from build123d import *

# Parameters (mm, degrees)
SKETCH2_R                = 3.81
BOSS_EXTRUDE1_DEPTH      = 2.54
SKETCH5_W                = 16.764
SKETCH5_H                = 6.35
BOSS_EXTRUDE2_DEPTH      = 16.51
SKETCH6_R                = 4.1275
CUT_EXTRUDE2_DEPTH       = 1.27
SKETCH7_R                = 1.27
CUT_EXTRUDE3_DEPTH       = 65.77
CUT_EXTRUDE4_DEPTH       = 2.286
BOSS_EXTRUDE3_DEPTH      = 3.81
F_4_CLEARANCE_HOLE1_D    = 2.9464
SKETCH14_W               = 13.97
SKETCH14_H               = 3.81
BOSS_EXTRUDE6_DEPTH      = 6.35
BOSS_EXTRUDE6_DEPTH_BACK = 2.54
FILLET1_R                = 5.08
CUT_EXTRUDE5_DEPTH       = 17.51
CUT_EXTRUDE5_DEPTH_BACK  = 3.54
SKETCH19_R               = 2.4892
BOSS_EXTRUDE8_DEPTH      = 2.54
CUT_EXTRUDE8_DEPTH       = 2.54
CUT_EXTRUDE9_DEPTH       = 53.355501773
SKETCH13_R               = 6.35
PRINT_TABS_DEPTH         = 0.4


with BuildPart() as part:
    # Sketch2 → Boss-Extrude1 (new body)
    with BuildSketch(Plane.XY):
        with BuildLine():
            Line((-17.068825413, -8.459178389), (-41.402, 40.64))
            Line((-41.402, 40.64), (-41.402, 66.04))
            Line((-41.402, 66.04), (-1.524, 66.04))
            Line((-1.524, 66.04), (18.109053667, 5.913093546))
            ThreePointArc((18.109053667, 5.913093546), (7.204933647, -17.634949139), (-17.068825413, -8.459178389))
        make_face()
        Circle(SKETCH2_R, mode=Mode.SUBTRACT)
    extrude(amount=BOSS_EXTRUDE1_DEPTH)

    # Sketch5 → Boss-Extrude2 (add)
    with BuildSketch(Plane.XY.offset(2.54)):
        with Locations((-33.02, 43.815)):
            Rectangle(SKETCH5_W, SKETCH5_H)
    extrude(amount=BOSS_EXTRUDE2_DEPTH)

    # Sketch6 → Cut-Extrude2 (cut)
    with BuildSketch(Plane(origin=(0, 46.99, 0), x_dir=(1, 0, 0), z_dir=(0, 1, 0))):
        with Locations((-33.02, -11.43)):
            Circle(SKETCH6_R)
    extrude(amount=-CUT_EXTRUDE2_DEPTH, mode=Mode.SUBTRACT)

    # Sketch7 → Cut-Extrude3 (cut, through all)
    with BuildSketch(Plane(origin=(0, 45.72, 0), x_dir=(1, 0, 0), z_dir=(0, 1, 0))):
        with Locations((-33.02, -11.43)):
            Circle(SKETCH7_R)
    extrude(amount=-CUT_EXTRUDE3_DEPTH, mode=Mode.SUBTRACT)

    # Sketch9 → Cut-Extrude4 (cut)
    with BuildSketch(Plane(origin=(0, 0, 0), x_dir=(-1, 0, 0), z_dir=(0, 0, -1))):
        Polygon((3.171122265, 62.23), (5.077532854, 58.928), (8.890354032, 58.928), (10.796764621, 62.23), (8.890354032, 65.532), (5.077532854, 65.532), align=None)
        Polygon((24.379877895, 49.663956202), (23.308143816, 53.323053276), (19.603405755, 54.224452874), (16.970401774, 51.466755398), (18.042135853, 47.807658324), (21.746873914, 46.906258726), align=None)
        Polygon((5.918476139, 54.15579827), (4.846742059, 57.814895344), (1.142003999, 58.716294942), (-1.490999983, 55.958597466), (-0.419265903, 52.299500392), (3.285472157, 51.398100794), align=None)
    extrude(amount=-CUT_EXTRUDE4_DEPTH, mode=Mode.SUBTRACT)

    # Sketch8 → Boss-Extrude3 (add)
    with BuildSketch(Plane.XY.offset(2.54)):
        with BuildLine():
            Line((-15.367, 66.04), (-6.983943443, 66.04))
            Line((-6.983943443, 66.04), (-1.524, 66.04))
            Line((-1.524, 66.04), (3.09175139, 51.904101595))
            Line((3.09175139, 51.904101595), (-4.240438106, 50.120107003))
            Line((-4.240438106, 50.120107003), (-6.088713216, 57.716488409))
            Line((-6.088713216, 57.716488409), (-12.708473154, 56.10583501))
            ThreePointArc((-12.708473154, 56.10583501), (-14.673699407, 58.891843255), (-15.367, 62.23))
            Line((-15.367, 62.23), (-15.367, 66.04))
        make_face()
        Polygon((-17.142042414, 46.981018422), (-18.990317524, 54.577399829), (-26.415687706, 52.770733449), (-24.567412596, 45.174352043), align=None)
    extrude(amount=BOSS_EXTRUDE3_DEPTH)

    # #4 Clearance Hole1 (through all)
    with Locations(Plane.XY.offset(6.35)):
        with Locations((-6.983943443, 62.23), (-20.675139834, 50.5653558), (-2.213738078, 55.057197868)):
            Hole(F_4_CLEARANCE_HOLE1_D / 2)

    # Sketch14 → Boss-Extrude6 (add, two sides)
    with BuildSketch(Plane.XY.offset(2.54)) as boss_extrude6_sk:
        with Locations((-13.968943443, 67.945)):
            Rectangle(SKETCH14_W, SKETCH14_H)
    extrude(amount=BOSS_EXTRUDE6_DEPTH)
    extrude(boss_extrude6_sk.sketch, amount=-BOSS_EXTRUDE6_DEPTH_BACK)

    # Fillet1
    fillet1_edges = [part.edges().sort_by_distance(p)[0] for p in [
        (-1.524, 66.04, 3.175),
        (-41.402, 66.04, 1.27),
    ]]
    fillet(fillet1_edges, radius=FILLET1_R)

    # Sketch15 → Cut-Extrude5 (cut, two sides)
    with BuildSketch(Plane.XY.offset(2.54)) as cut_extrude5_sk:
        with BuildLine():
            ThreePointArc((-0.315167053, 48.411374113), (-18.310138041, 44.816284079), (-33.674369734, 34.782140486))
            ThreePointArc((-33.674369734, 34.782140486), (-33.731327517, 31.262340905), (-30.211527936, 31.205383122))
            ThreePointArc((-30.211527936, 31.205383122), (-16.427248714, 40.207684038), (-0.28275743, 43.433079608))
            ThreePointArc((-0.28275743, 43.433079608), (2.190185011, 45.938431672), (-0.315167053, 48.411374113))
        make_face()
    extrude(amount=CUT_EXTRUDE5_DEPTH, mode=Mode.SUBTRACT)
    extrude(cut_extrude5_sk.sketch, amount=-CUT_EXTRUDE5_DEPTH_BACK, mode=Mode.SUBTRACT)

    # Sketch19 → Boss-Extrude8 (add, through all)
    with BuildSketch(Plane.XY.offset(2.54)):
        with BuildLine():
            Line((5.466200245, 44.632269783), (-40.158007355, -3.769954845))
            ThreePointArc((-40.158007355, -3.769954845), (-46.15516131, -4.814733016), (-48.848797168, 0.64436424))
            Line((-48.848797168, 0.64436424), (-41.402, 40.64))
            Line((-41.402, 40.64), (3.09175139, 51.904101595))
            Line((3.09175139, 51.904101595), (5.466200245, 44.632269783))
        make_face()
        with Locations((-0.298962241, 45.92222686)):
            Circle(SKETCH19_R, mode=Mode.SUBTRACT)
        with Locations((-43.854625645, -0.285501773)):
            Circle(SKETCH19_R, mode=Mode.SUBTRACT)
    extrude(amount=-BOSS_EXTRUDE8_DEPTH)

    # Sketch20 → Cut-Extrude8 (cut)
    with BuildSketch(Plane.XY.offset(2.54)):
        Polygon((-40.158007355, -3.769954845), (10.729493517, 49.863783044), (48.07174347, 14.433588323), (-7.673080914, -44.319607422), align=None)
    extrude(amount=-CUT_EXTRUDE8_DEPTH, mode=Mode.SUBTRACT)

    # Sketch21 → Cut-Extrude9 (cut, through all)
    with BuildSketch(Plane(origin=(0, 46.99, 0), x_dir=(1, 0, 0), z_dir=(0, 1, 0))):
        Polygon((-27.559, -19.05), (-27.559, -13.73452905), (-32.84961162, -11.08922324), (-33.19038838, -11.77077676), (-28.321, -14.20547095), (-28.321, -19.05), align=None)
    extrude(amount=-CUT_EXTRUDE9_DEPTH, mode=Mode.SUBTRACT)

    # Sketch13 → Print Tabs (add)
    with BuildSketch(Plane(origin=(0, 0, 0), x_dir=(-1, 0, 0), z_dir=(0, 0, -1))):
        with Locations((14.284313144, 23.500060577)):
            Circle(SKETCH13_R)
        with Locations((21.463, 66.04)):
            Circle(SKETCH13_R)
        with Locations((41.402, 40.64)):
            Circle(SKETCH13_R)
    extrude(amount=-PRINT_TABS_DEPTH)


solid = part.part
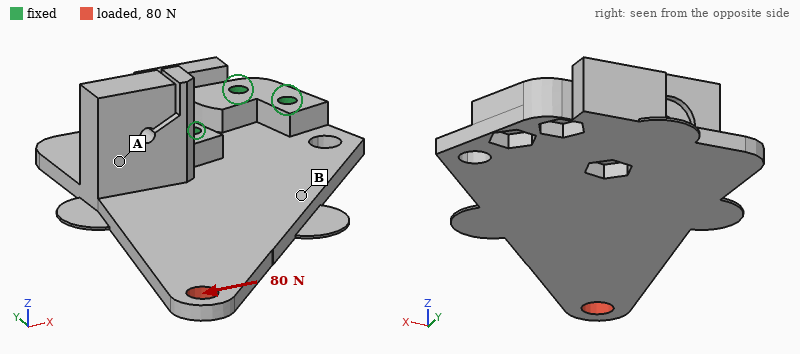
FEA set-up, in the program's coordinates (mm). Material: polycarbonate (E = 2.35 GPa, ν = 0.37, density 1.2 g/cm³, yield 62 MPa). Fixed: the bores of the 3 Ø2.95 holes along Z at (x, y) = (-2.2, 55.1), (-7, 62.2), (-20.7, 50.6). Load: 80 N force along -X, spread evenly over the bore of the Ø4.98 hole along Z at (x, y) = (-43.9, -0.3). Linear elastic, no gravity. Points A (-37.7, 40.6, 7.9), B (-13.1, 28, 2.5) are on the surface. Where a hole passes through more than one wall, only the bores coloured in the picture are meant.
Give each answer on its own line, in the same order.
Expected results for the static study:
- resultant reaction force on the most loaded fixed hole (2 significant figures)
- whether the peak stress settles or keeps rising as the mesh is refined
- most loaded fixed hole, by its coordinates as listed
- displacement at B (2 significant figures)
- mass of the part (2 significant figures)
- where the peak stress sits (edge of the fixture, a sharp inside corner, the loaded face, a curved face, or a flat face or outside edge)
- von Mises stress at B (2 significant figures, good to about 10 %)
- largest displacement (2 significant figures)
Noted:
190 N
keeps rising
(-20.7, 50.6)
0.19 mm
10 g
edge of the fixture
5.5 MPa
0.78 mm
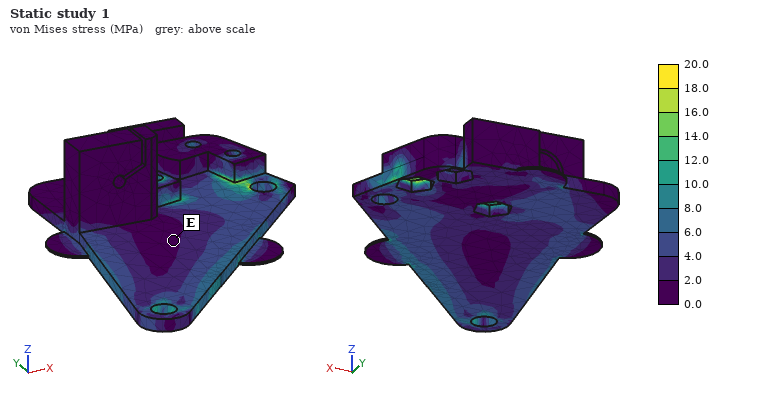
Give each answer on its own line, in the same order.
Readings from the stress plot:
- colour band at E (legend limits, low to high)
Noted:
0.0 to 2.0 MPa
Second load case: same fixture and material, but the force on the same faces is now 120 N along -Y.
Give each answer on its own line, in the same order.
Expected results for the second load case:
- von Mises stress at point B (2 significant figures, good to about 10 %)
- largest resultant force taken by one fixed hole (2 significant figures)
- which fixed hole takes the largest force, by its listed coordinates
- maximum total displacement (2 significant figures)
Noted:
3.1 MPa
190 N
(-20.7, 50.6)
0.75 mm
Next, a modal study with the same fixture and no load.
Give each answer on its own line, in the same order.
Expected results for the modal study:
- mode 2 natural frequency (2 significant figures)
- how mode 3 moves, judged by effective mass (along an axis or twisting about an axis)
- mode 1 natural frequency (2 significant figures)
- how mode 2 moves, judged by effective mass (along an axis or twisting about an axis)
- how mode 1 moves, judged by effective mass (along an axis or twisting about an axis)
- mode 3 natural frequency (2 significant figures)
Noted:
980 Hz
along Z
310 Hz
twisting about Y
along Z
1100 Hz
